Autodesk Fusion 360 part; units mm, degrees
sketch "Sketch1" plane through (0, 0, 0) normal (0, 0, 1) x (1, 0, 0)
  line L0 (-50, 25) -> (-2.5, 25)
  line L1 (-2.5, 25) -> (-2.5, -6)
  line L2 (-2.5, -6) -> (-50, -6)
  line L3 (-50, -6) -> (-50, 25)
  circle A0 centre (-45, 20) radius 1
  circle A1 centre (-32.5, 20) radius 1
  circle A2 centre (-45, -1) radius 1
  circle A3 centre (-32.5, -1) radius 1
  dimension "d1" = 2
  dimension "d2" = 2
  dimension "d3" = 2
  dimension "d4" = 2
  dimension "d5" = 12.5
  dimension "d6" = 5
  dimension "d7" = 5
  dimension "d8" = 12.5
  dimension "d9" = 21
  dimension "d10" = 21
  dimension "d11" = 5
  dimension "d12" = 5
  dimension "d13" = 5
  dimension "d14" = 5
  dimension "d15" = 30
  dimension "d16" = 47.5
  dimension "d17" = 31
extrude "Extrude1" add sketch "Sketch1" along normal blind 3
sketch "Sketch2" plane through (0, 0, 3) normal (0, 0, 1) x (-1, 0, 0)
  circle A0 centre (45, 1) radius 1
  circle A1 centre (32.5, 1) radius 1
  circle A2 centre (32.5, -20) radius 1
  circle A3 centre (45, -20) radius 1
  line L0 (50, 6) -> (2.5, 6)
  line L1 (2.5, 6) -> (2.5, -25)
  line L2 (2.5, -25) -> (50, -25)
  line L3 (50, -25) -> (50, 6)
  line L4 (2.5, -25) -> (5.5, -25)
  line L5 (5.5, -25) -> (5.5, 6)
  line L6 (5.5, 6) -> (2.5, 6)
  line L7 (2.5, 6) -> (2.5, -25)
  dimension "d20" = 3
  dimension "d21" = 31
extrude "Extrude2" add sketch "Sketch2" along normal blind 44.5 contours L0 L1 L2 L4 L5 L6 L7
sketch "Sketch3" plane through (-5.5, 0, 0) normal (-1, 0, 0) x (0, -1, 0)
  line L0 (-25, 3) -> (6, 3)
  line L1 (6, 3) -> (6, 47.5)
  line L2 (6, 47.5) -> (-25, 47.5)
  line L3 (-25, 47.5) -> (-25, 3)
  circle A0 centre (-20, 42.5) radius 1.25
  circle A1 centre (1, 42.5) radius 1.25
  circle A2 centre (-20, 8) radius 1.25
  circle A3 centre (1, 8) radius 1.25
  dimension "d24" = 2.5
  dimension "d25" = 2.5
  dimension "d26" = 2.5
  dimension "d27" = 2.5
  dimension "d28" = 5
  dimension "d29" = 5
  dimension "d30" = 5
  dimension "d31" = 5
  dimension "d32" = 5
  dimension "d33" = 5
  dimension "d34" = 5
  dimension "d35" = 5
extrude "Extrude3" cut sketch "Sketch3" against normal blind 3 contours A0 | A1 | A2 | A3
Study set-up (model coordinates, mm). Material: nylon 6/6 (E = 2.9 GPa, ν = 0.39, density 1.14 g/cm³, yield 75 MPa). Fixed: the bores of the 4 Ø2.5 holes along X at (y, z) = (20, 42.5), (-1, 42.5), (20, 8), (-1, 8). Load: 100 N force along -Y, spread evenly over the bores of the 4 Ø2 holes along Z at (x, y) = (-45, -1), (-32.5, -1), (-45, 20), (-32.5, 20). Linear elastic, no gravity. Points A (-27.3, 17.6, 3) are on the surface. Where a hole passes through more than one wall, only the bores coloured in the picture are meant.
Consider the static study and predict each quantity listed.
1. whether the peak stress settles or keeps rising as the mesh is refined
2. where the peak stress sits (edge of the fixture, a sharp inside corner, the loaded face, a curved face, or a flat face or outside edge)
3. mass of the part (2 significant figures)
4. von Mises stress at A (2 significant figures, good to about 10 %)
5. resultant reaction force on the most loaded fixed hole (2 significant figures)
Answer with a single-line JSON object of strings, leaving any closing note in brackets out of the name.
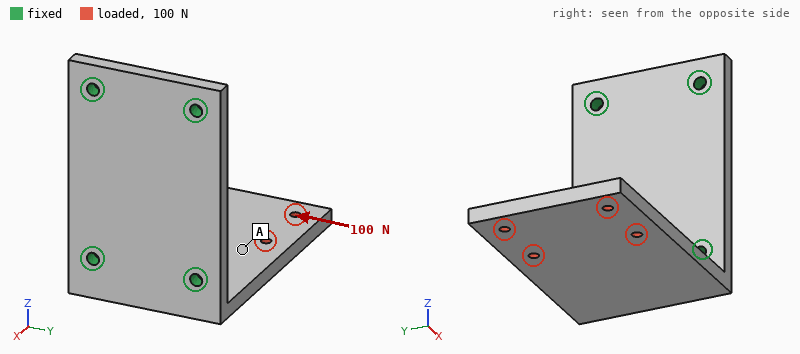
{"whether the peak stress settles or keeps rising as the mesh is refined": "keeps rising", "where the peak stress sits": "edge of the fixture", "mass of the part": "9.6 g", "von Mises stress at A": "3.4 MPa", "resultant reaction force on the most loaded fixed hole": "170 N"}
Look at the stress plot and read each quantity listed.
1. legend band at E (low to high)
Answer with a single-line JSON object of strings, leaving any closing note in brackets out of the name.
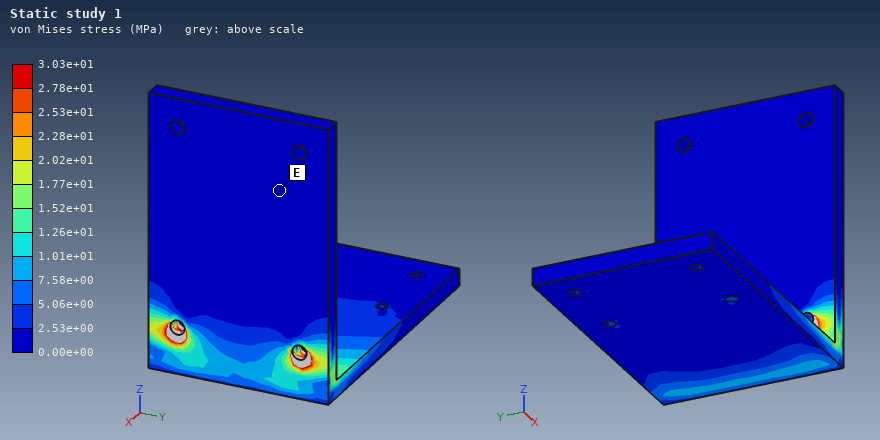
{"legend band at E": "0.00e+00 to 2.53e+00 MPa"}
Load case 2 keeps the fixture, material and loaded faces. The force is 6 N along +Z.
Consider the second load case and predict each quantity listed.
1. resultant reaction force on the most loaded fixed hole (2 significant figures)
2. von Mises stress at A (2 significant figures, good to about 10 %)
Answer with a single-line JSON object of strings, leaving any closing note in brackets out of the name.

{"resultant reaction force on the most loaded fixed hole": "2.9 N", "von Mises stress at A": "1.4 MPa"}
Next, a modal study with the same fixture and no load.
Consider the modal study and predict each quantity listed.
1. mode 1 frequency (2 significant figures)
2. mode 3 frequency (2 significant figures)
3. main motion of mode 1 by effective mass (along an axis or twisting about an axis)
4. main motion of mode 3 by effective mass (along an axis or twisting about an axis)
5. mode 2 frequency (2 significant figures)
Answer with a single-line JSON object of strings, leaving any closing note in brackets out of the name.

{"mode 1 frequency": "310 Hz", "mode 3 frequency": "1400 Hz", "main motion of mode 1 by effective mass": "along Z", "main motion of mode 3 by effective mass": "along Y", "mode 2 frequency": "1000 Hz"}
